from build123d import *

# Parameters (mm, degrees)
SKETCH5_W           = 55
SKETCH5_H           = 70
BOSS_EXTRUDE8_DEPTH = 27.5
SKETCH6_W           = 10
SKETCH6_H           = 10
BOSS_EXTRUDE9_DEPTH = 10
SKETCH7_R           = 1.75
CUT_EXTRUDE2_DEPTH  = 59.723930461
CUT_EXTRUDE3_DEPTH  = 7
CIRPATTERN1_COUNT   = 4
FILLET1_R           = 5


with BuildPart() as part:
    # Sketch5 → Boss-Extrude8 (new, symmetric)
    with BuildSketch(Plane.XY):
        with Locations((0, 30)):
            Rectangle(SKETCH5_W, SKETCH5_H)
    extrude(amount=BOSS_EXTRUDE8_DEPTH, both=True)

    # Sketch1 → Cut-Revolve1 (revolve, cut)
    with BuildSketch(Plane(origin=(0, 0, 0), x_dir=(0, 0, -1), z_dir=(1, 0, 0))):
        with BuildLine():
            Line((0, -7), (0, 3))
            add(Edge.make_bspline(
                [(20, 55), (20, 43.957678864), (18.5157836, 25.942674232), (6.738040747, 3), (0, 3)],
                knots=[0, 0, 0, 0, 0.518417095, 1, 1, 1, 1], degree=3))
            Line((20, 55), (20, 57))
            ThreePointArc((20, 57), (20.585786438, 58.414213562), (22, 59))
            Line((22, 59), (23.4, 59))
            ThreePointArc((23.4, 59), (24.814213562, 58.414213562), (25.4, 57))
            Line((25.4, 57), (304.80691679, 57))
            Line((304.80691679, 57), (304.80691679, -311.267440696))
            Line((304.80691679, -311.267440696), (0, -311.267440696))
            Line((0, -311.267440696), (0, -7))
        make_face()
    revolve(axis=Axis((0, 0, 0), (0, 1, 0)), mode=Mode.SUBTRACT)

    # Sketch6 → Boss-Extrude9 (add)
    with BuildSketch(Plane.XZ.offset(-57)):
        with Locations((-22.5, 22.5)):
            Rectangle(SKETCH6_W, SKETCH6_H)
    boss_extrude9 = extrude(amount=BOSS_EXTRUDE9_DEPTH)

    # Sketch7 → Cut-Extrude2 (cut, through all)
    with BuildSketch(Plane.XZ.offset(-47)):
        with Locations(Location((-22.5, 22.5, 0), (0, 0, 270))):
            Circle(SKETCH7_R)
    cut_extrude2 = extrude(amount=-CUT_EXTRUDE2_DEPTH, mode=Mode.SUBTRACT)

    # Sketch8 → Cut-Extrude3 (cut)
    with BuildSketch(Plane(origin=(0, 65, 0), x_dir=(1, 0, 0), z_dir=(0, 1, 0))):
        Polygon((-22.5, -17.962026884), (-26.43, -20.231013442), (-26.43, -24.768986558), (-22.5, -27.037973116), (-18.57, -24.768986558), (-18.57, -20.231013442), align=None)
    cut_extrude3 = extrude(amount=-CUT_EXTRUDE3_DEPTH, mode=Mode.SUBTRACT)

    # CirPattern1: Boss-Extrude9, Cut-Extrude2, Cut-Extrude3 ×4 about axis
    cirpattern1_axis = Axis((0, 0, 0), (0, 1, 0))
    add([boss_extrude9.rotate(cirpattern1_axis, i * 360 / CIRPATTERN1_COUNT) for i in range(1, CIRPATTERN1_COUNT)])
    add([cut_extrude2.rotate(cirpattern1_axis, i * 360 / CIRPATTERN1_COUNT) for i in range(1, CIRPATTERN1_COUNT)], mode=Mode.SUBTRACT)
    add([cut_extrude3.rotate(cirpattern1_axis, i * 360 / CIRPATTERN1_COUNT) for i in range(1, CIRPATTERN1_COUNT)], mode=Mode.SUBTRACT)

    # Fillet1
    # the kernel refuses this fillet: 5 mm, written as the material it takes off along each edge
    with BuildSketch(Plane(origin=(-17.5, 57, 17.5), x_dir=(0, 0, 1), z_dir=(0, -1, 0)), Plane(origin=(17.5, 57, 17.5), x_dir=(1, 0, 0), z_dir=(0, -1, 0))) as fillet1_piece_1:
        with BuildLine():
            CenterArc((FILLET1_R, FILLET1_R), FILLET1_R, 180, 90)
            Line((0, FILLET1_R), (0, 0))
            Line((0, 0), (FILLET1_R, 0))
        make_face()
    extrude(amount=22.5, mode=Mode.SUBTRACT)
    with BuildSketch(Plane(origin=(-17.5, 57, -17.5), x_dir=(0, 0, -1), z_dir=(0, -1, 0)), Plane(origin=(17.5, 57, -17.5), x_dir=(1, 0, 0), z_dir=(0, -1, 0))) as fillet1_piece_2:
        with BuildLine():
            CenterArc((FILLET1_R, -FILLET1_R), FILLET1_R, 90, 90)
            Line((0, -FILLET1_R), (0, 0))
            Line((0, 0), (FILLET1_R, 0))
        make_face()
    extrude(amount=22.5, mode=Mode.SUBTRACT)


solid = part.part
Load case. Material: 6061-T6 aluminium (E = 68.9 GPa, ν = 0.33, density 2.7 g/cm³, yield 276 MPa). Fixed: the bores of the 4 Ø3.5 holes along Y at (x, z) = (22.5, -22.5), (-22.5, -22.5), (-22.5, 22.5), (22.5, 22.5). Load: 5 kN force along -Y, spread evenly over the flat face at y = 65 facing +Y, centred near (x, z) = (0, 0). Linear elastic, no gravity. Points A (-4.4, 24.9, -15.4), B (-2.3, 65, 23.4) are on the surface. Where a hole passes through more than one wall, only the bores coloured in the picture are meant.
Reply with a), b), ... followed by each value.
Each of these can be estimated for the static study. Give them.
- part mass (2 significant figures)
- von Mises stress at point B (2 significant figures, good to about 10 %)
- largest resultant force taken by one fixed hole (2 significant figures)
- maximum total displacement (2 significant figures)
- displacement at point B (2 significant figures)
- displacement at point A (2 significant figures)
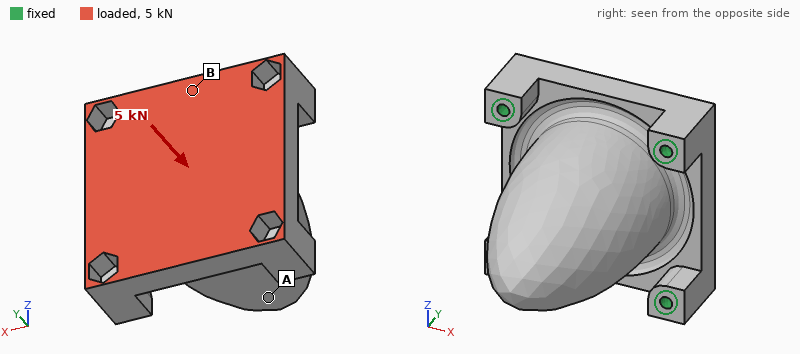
a) 190 g
b) 18 MPa
c) 1.5 kN
d) 14 µm
e) 12 µm
f) 13 µm
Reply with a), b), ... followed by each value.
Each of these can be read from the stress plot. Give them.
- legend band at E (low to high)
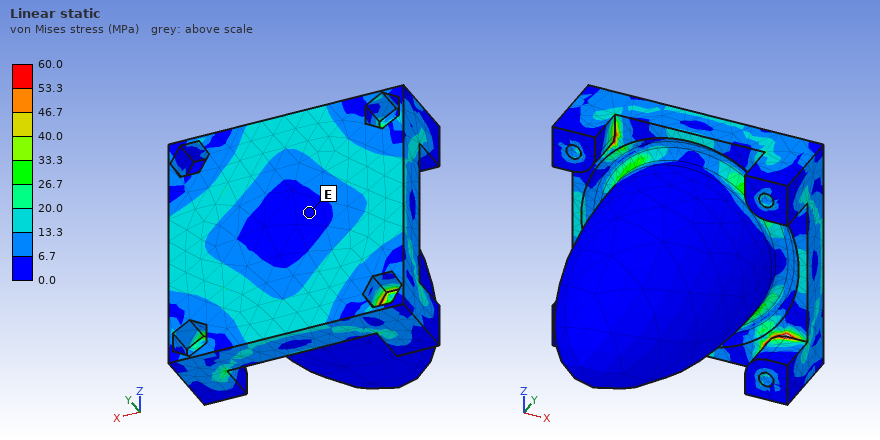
a) 0.0 to 6.7 MPa
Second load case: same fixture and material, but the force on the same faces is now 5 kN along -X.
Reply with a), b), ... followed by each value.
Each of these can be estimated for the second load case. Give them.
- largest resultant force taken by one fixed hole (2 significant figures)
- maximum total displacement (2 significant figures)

a) 1.3 kN
b) 12 µm
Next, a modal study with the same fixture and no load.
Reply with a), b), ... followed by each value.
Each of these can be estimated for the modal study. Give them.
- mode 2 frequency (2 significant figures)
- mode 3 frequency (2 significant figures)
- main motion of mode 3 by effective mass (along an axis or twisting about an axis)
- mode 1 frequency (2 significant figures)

a) 4000 Hz
b) 6600 Hz
c) along Y
d) 4000 Hz
